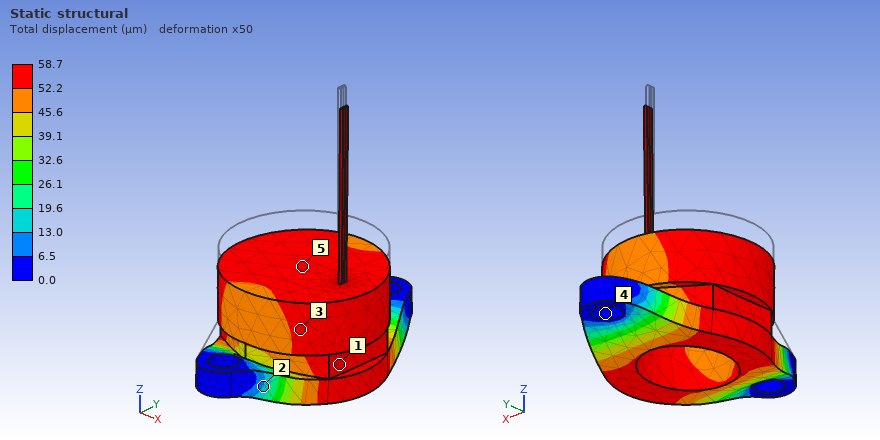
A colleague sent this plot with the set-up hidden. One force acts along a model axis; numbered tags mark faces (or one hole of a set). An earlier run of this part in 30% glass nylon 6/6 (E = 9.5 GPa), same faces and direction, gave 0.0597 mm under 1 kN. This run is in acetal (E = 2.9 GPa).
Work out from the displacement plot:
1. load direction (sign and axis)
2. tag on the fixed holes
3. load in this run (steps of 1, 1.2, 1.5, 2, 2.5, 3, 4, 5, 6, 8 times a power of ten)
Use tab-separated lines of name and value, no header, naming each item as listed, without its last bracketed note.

load direction	-Z
tag on the fixed holes	4
load in this run	300 N
